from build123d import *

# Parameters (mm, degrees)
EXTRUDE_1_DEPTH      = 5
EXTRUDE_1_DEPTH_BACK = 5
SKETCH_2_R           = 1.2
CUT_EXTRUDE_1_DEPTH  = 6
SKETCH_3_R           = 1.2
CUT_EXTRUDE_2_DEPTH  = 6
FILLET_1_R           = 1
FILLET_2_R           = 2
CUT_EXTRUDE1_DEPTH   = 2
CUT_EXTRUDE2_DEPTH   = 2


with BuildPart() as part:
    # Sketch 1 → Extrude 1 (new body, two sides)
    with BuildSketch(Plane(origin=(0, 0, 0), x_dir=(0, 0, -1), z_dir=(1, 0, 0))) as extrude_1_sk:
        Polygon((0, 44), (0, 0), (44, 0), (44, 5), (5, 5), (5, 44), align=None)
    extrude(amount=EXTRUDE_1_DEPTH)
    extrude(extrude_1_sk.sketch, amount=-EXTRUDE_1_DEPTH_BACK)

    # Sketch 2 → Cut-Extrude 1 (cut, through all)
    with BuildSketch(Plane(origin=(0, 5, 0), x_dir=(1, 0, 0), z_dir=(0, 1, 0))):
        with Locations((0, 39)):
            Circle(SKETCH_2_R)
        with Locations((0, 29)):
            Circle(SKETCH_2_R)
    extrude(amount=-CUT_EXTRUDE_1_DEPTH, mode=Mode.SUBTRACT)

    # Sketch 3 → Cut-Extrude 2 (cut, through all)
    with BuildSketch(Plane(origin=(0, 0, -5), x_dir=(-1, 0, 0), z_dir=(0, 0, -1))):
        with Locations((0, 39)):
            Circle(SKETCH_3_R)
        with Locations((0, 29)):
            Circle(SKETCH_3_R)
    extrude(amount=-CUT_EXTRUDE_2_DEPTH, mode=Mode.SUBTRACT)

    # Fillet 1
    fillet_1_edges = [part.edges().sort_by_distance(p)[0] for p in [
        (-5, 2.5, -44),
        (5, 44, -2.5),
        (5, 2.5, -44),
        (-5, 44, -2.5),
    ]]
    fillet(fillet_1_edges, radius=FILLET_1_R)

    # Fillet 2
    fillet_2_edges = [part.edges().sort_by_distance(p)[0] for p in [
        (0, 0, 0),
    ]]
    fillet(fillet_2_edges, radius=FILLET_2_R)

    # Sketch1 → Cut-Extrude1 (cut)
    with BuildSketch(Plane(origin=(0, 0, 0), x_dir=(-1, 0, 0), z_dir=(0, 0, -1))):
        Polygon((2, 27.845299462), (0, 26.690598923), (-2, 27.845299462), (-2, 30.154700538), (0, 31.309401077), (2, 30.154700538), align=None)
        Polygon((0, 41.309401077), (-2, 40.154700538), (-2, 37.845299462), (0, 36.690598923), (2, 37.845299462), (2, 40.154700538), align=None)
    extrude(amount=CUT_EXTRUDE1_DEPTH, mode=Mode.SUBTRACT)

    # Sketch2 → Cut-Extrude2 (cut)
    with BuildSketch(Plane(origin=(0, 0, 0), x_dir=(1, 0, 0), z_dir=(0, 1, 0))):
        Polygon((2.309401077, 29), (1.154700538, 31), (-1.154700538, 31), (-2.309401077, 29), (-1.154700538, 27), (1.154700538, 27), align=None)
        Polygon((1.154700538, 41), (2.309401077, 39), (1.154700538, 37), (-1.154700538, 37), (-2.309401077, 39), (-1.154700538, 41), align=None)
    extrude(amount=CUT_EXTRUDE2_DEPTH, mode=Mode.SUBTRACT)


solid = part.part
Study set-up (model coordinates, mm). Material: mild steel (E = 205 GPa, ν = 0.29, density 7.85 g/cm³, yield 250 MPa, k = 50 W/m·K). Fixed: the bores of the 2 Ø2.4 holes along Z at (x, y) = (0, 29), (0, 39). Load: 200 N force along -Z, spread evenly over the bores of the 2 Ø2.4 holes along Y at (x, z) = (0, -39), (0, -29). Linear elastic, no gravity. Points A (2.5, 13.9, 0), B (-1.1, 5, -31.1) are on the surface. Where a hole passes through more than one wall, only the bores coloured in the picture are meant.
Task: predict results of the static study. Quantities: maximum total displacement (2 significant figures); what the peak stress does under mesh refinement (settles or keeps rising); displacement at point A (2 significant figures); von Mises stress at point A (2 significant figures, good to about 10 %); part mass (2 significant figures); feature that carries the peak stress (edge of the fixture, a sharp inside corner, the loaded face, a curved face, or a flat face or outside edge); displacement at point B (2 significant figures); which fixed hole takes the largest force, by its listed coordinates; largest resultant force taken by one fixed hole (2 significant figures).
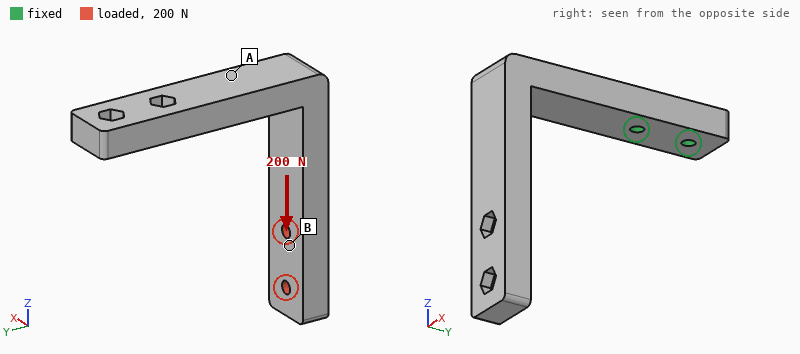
0.17 mm
keeps rising
0.033 mm
50 MPa
31 g
edge of the fixture
0.12 mm
(0, 29)
580 N
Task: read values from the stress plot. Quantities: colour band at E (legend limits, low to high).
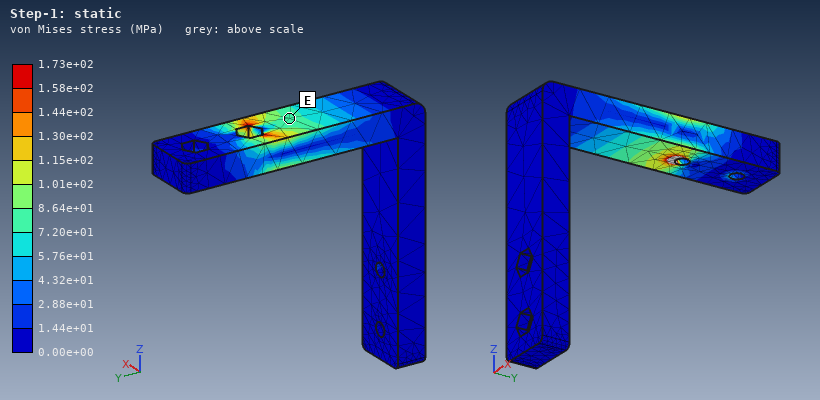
7.20e+01 to 8.64e+01 MPa
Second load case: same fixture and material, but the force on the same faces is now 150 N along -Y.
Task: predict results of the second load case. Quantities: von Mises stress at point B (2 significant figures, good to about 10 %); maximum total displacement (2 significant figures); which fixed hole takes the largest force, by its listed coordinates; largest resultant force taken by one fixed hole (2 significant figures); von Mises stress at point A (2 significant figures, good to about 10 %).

17 MPa
0.38 mm
(0, 29)
490 N
110 MPa
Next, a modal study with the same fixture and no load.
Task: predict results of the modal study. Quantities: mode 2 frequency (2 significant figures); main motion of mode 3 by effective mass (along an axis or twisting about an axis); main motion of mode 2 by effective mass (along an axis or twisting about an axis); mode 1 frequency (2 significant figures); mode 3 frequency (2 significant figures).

1400 Hz
along Z
along X
1100 Hz
3300 Hz
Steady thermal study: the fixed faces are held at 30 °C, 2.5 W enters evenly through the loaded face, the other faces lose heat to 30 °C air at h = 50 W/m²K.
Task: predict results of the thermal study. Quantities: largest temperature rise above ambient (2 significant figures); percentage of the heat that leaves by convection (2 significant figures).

30 K
64 %
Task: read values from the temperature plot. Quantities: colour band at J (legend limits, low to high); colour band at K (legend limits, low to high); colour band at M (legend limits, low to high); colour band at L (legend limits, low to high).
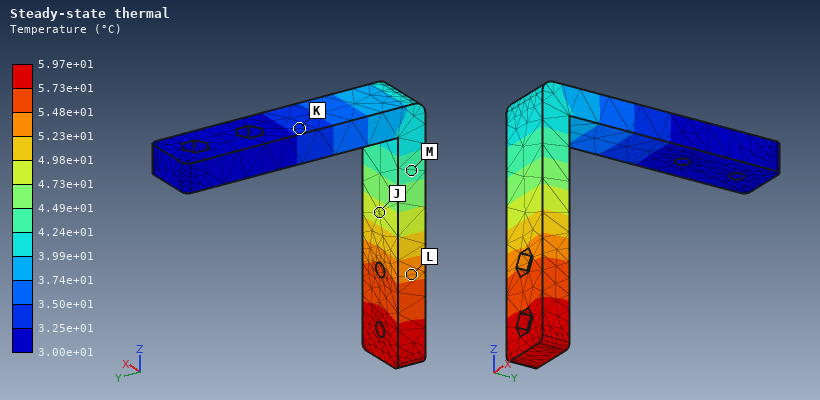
4.73e+01 to 4.98e+01 °C
3.25e+01 to 3.50e+01 °C
4.24e+01 to 4.49e+01 °C
5.23e+01 to 5.48e+01 °C
